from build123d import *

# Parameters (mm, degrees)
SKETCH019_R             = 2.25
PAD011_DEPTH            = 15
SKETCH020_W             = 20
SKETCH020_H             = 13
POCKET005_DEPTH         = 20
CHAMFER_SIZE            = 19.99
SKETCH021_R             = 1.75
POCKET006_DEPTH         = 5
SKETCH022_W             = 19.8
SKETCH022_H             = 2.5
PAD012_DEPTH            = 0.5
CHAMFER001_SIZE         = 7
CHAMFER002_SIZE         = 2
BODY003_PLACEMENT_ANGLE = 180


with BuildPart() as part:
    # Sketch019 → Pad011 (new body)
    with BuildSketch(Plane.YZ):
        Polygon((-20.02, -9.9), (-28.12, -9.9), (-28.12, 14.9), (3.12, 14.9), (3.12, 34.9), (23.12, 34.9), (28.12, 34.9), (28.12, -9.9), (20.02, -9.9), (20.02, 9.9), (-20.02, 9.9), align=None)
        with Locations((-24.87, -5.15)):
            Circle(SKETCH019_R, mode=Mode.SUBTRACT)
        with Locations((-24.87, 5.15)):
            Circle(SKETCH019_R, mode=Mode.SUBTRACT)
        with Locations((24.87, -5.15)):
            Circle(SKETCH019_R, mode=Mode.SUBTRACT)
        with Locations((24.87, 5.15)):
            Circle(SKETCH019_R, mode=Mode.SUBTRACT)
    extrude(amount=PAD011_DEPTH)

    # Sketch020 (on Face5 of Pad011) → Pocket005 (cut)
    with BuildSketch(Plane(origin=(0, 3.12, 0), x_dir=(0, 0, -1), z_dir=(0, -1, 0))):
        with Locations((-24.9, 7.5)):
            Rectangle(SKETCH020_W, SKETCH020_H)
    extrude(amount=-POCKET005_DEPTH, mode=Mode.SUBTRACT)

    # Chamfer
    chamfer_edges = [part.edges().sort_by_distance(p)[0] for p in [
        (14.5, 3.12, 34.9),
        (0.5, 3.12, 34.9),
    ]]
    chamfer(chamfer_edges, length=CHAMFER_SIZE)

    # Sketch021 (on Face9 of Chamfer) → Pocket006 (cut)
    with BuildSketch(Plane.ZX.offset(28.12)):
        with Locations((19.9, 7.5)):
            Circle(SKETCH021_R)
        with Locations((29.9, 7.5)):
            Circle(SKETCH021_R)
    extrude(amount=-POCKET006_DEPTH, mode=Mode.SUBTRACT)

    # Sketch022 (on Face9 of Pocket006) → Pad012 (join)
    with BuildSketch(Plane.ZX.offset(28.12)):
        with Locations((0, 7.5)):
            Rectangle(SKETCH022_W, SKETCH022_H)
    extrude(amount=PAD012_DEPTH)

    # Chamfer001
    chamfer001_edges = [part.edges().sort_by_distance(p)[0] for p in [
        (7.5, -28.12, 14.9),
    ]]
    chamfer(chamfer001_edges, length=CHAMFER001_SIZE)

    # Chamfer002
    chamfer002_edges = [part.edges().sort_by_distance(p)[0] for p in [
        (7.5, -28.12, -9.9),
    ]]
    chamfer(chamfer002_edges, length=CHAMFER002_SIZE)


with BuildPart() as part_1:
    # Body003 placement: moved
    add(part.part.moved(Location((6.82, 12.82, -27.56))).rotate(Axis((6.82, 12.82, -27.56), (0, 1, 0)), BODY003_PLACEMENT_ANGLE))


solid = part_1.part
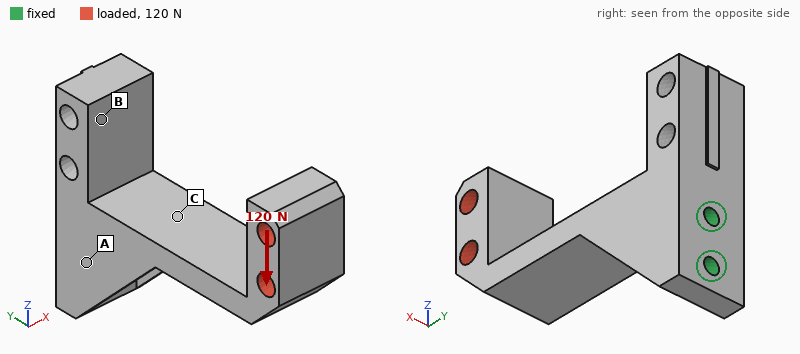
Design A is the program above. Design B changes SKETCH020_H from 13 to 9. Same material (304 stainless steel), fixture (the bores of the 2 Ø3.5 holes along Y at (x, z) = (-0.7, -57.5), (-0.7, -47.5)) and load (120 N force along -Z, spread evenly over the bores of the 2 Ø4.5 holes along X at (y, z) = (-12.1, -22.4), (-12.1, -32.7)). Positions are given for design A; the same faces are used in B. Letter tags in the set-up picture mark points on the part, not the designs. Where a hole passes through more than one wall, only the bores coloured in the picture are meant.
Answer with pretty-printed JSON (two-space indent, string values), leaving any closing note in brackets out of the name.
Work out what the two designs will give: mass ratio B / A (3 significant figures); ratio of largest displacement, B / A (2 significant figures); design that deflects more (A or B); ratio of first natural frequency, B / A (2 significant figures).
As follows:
{
  "mass ratio B / A": "1.08",
  "ratio of largest displacement, B / A": "0.80",
  "design that deflects more": "A",
  "ratio of first natural frequency, B / A": "1.1"
}
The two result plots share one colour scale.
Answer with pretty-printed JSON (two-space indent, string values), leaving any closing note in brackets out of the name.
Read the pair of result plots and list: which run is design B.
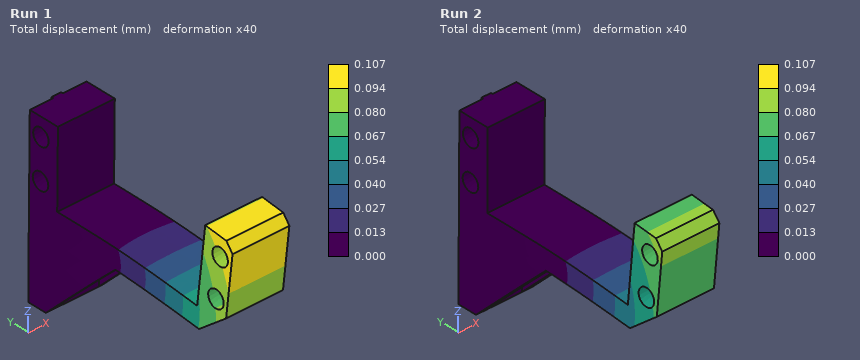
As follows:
{
  "which run is design B": "Run 2"
}
